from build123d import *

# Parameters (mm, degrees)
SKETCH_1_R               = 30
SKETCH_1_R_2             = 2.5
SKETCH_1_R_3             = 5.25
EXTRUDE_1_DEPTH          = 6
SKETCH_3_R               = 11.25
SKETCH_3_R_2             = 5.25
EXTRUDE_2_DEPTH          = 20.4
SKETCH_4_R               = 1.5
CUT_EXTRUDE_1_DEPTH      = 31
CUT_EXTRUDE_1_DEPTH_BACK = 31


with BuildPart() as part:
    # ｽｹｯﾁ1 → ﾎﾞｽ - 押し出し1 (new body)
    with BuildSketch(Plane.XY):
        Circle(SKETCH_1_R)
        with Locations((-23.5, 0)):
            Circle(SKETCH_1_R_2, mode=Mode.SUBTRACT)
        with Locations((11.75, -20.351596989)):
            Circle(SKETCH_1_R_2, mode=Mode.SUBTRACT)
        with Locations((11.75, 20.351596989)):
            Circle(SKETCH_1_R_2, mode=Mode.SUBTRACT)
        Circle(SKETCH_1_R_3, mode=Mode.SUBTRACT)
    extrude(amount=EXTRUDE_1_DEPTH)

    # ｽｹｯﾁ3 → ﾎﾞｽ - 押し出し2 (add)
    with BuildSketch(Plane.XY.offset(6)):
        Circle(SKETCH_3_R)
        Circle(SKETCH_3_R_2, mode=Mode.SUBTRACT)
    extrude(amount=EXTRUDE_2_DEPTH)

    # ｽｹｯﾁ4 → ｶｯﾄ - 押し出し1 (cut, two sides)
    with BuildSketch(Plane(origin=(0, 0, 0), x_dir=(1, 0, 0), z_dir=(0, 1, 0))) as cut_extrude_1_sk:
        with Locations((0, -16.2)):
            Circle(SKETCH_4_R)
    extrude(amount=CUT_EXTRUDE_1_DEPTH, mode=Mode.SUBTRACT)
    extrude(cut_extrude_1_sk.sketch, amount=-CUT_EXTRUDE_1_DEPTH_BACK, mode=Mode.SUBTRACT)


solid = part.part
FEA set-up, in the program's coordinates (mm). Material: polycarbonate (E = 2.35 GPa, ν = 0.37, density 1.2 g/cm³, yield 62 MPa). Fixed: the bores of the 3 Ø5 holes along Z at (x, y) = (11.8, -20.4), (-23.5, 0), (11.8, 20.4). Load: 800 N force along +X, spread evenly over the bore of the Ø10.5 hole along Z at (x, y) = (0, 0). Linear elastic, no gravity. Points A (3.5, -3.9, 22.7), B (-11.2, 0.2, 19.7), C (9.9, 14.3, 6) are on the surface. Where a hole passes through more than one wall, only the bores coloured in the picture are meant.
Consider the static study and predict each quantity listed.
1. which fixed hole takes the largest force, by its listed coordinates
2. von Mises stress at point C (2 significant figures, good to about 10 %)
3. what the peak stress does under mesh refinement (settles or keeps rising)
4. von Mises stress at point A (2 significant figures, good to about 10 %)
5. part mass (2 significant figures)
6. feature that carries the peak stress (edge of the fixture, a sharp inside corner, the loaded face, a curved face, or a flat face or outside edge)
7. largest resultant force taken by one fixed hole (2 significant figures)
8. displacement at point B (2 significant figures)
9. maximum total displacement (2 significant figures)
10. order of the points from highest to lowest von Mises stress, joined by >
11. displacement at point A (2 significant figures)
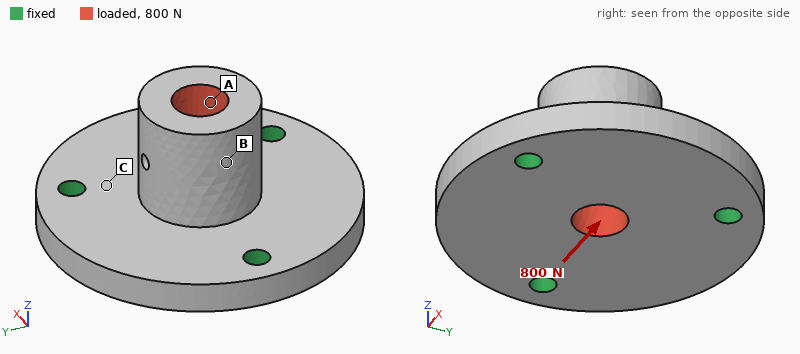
(-23.5, 0)
4.4 MPa
keeps rising
2.2 MPa
27 g
edge of the fixture
400 N
0.20 mm
0.26 mm
C > A > B
0.21 mm
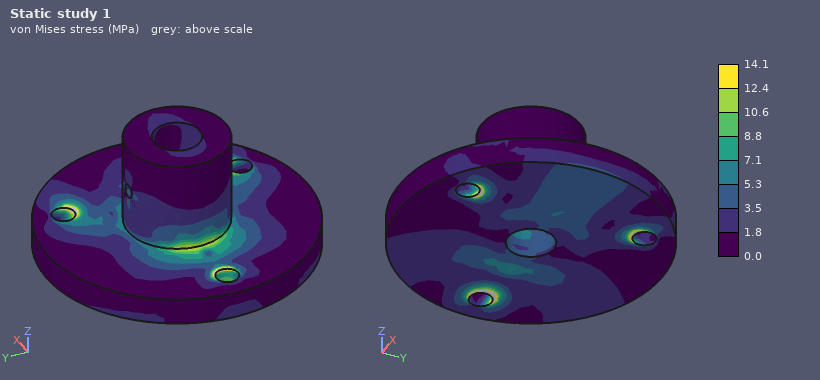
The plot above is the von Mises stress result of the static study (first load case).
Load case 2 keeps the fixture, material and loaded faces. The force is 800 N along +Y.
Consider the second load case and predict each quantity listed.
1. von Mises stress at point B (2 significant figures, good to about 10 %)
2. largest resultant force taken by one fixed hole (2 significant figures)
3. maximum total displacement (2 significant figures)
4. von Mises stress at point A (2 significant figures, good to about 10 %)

1.7 MPa
360 N
0.25 mm
2.4 MPa
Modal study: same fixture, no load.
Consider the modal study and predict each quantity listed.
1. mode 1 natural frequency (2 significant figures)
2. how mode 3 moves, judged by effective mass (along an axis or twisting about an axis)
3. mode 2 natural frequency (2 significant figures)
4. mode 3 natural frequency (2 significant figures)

2800 Hz
along Z
2800 Hz
3200 Hz
